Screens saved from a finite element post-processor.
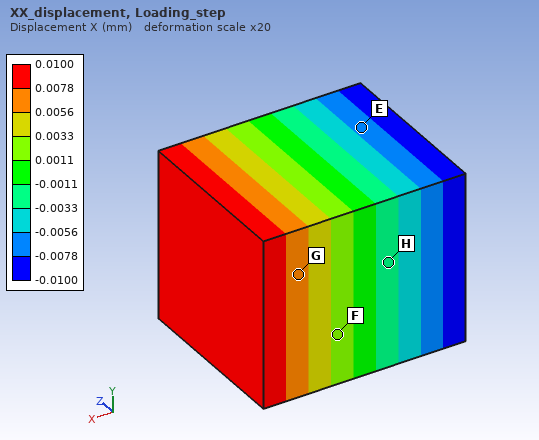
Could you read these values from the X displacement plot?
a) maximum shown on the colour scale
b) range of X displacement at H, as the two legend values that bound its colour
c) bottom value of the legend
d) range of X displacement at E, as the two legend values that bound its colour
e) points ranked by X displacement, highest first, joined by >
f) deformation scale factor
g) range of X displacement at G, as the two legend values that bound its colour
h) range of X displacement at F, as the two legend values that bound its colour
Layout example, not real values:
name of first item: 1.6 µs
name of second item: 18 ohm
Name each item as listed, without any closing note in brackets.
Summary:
maximum shown on the colour scale: 0.0100 mm
range of X displacement at H, as the two legend values that bound its colour: -0.0033 to -0.0011 mm
bottom value of the legend: -0.0100 mm
range of X displacement at E, as the two legend values that bound its colour: -0.0078 to -0.0056 mm
points ranked by X displacement, highest first, joined by >: G > F > H > E
deformation scale factor: 20
range of X displacement at G, as the two legend values that bound its colour: 0.0056 to 0.0078 mm
range of X displacement at F, as the two legend values that bound its colour: 0.0011 to 0.0033 mm
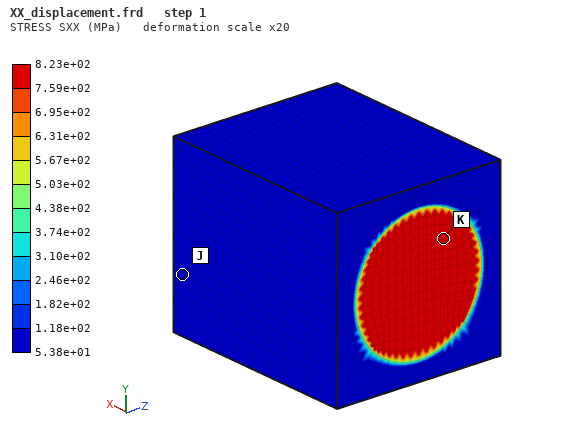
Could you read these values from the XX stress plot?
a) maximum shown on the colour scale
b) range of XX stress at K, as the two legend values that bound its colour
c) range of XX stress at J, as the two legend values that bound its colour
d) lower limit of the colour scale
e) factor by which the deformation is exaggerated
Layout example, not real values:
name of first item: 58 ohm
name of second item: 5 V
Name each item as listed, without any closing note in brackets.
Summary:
maximum shown on the colour scale: 8.23e+02 MPa
range of XX stress at K, as the two legend values that bound its colour: 7.59e+02 to 8.23e+02 MPa
range of XX stress at J, as the two legend values that bound its colour: 5.38e+01 to 1.18e+02 MPa
lower limit of the colour scale: 5.38e+01 MPa
factor by which the deformation is exaggerated: 20
